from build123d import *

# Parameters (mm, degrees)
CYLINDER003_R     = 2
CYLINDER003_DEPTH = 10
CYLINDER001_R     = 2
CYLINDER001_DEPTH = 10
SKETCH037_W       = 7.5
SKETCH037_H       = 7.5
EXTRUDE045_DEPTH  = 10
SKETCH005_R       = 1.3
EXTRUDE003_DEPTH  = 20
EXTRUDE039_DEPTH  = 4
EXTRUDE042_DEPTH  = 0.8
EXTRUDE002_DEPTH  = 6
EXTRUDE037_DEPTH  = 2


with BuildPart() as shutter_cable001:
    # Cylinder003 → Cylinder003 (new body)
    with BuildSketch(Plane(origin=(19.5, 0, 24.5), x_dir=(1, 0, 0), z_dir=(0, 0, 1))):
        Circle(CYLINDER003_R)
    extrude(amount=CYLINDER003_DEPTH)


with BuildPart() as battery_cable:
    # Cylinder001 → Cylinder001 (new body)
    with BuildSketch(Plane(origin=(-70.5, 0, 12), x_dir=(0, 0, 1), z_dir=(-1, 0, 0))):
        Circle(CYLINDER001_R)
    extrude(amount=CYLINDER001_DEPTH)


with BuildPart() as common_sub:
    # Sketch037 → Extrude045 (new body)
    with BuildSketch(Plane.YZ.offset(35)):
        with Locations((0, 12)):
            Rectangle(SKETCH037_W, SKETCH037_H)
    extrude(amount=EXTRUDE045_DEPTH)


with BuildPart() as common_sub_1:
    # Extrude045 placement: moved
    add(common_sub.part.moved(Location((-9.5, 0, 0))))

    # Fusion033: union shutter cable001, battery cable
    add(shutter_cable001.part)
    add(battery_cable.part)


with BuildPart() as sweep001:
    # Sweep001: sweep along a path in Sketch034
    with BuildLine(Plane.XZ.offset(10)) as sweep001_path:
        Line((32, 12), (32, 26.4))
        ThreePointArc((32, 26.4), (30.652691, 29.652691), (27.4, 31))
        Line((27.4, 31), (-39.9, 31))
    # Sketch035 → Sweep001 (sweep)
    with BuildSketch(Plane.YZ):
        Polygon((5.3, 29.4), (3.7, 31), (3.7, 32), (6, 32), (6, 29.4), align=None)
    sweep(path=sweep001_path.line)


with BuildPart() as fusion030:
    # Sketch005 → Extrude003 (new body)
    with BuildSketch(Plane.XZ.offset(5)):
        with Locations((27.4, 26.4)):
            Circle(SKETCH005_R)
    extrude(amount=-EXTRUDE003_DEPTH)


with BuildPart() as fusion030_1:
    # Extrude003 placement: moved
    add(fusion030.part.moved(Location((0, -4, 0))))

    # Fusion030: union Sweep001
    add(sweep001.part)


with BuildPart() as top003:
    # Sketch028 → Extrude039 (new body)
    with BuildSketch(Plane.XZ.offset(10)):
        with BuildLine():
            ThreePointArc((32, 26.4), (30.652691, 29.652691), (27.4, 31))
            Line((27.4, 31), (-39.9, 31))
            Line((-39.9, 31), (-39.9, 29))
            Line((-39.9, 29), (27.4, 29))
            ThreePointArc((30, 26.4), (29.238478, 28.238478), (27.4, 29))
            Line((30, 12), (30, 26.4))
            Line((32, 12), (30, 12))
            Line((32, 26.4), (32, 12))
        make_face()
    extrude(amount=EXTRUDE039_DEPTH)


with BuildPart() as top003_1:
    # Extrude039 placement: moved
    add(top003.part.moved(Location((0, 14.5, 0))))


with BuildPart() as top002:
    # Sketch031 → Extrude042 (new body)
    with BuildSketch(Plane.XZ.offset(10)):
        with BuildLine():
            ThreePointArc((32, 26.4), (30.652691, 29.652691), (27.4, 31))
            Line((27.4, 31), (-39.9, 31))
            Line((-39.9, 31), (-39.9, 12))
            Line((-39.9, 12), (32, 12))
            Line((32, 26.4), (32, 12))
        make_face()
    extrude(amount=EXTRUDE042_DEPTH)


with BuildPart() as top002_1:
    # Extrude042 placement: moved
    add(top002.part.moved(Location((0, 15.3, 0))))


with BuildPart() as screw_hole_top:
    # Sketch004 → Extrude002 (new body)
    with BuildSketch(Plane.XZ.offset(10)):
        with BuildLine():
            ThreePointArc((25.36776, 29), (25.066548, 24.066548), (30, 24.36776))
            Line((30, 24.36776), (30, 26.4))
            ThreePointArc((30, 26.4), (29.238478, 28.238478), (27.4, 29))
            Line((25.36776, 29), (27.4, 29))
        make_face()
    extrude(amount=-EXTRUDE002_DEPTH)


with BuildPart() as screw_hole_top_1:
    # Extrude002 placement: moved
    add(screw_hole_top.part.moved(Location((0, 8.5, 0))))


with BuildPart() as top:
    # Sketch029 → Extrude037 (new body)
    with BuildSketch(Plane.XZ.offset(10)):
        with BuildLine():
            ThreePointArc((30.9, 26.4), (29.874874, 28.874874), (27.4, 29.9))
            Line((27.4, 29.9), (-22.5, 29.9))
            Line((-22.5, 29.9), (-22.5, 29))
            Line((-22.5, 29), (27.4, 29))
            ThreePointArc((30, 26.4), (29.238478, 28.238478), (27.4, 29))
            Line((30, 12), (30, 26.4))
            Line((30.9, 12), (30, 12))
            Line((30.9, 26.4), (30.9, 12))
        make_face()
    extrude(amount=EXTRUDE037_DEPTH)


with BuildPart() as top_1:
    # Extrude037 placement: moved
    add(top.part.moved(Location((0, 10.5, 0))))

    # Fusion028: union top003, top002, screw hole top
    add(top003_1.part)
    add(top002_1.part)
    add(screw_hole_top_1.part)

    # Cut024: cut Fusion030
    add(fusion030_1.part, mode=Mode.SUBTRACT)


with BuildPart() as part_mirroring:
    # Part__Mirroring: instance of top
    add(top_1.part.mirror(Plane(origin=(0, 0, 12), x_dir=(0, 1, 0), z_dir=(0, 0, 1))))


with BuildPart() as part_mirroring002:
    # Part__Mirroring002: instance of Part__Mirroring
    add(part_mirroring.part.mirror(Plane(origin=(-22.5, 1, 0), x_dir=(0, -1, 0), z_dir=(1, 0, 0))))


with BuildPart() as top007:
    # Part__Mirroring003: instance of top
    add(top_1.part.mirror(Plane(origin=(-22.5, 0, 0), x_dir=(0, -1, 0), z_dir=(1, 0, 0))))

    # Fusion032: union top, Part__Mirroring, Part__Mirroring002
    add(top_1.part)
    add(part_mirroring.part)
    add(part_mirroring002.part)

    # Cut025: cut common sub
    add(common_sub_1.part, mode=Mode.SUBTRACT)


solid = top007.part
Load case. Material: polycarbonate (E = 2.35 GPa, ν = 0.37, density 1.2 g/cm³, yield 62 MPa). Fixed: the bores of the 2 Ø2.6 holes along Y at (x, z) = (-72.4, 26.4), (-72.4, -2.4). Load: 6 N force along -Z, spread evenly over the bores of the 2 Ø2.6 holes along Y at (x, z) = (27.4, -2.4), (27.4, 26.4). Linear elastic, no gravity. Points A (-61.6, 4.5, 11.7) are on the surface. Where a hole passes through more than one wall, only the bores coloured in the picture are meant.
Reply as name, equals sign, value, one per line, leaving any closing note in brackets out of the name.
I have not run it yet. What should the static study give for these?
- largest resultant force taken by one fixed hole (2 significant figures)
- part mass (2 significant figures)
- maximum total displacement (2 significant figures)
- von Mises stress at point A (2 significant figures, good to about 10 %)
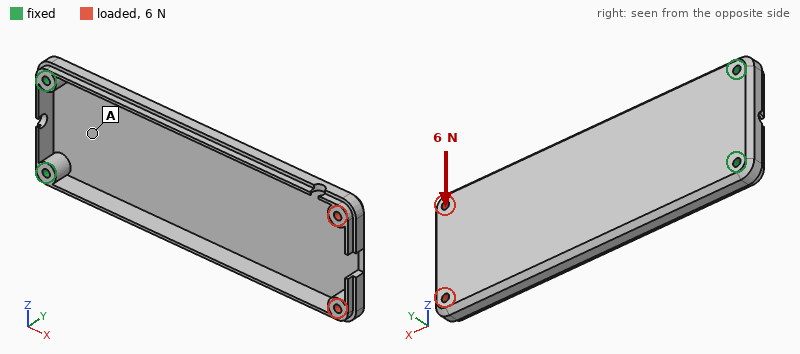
largest resultant force taken by one fixed hole = 20 N
part mass = 7.4 g
maximum total displacement = 1.2 mm
von Mises stress at point A = 0.50 MPa
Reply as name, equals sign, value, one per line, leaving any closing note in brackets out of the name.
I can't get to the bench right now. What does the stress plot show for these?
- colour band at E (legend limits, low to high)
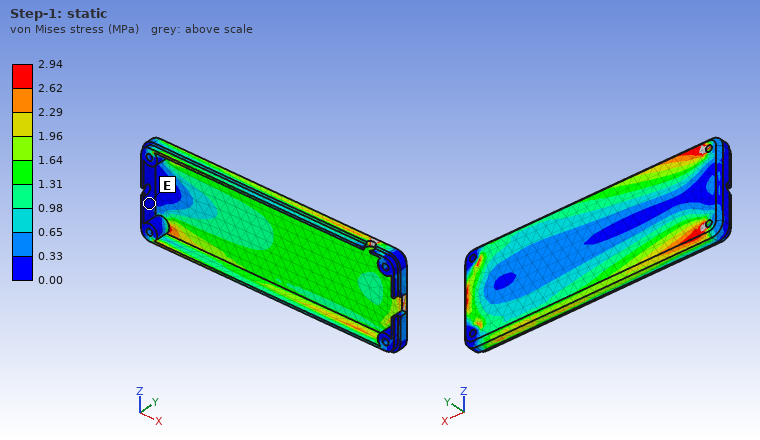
colour band at E = 0.00 to 0.33 MPa
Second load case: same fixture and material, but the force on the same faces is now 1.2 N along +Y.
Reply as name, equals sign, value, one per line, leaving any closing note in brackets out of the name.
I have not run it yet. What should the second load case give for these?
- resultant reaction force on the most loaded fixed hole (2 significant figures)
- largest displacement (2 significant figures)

resultant reaction force on the most loaded fixed hole = 2.1 N
largest displacement = 1.4 mm
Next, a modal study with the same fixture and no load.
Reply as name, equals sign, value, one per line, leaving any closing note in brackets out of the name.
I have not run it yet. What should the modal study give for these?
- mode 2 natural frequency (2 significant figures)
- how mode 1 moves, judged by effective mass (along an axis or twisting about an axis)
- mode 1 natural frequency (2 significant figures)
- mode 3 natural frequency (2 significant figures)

mode 2 natural frequency = 170 Hz
how mode 1 moves, judged by effective mass = along Y
mode 1 natural frequency = 100 Hz
mode 3 natural frequency = 520 Hz
